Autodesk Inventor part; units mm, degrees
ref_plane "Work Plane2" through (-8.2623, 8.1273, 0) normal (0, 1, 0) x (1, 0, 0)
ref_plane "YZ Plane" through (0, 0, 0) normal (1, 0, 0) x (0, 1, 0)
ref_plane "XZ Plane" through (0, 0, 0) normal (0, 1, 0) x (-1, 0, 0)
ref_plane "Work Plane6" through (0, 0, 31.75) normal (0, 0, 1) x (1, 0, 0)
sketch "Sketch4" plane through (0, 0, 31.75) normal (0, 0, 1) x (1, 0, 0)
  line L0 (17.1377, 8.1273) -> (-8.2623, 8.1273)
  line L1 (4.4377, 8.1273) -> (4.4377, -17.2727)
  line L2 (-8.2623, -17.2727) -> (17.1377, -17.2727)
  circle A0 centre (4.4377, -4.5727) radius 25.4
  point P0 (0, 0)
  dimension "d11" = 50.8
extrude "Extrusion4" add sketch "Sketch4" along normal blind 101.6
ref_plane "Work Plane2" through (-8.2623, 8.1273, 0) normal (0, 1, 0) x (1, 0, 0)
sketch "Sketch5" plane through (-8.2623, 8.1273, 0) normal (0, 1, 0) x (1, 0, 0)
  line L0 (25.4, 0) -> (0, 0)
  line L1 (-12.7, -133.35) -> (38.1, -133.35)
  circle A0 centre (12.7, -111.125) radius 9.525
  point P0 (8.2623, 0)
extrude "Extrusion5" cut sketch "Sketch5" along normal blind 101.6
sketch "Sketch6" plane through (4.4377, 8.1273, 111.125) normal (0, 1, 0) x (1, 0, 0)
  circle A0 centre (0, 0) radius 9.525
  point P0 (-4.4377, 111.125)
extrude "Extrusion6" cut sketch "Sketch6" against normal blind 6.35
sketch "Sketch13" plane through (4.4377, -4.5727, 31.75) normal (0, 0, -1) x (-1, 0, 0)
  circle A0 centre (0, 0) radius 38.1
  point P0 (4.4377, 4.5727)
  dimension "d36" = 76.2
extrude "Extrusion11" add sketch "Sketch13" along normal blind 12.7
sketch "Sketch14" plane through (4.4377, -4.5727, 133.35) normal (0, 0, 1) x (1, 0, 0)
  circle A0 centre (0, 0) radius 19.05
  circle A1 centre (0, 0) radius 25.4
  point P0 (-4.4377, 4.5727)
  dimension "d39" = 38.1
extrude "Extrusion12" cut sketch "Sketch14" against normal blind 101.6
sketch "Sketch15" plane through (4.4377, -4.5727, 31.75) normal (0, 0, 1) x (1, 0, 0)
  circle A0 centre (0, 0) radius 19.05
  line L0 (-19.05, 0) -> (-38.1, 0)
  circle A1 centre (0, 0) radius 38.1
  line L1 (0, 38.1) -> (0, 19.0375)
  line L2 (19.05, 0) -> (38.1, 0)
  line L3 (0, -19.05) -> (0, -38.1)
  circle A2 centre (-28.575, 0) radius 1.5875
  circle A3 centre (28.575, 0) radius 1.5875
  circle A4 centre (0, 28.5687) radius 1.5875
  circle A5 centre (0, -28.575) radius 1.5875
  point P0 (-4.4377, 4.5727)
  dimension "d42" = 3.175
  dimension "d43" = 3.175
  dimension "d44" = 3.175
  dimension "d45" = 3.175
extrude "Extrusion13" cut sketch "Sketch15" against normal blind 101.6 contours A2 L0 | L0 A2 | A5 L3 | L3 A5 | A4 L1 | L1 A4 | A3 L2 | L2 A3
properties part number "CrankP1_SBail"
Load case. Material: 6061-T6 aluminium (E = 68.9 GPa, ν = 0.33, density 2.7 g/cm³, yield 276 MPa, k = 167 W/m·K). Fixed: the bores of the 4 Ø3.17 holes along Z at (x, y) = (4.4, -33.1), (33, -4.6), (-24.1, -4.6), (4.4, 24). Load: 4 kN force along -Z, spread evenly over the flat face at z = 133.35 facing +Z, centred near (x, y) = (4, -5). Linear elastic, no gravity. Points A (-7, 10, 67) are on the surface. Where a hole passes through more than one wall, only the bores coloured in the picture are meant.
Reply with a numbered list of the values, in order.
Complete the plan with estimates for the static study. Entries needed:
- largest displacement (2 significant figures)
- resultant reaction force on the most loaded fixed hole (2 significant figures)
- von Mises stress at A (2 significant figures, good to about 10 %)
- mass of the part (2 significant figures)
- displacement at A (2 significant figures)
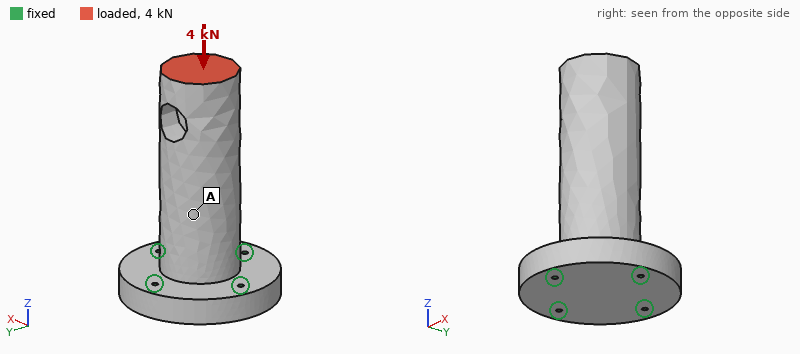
1. 12 µm
2. 1.0 kN
3. 3.4 MPa
4. 460 g
5. 5.3 µm
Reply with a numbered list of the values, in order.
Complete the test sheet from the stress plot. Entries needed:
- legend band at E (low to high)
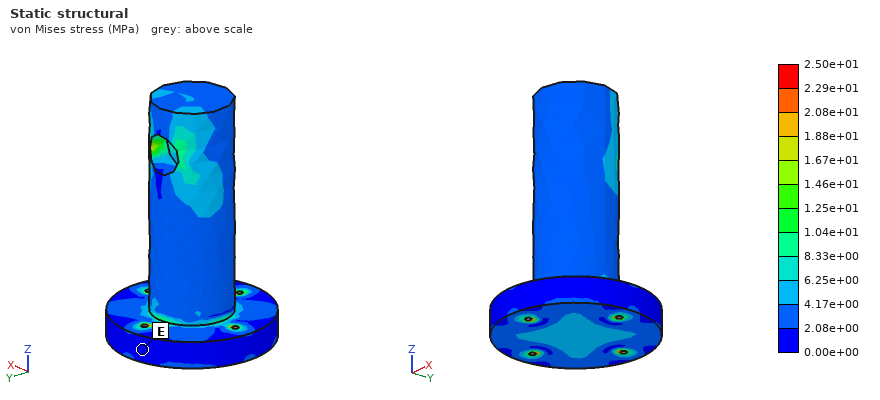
1. 0.00e+00 to 2.08e+00 MPa
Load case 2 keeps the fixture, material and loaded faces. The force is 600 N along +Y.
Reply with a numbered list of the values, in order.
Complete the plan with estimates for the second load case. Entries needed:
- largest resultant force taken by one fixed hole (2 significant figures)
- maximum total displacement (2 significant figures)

1. 1.1 kN
2. 53 µm
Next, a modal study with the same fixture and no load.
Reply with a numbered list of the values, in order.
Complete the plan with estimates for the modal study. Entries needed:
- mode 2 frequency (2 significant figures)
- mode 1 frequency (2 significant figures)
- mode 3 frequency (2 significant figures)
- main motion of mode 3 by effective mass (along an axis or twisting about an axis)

1. 1900 Hz
2. 1900 Hz
3. 7300 Hz
4. twisting about Z
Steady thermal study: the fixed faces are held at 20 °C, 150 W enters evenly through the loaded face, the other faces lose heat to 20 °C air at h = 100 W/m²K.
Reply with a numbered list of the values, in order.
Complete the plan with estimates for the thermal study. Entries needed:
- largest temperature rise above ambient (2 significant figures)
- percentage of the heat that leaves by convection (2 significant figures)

1. 76 K
2. 37 %
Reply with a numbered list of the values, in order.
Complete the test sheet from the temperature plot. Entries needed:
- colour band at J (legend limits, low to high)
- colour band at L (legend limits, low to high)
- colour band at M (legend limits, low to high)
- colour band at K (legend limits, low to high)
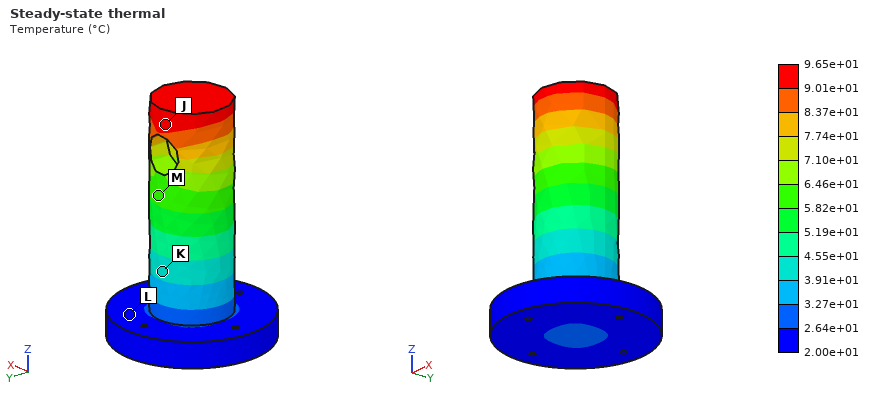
1. 9.01e+01 to 9.65e+01 °C
2. 2.00e+01 to 2.64e+01 °C
3. 5.82e+01 to 6.46e+01 °C
4. 3.91e+01 to 4.55e+01 °C
